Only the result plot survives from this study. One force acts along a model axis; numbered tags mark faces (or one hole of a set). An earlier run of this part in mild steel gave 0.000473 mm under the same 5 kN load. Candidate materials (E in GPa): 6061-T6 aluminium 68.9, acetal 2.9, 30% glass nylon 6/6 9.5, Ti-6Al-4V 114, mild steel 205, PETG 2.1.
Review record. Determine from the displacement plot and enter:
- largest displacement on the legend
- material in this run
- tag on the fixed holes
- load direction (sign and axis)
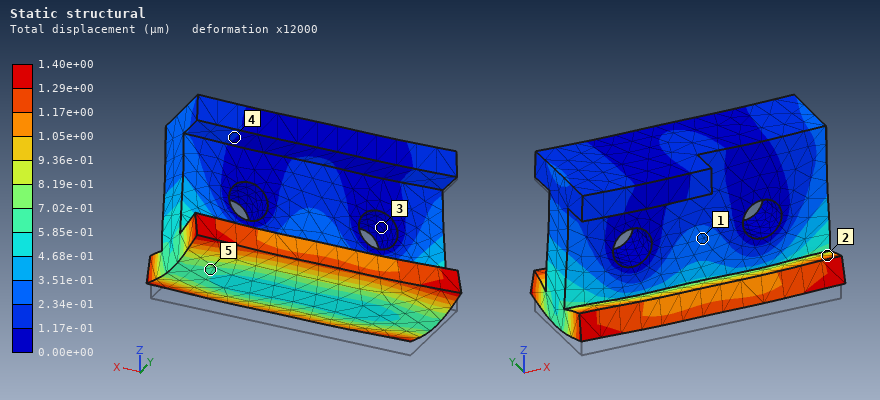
1.40e+00 µm
6061-T6 aluminium
3
+Z
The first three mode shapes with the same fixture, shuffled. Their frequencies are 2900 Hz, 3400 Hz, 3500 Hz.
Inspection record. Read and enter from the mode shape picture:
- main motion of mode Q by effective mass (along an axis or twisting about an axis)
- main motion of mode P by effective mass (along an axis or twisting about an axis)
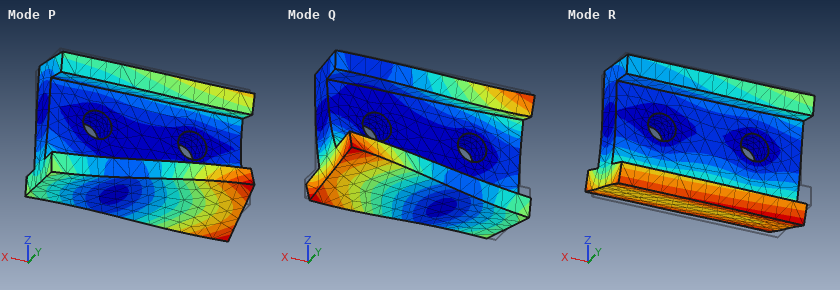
along Y
along Y
